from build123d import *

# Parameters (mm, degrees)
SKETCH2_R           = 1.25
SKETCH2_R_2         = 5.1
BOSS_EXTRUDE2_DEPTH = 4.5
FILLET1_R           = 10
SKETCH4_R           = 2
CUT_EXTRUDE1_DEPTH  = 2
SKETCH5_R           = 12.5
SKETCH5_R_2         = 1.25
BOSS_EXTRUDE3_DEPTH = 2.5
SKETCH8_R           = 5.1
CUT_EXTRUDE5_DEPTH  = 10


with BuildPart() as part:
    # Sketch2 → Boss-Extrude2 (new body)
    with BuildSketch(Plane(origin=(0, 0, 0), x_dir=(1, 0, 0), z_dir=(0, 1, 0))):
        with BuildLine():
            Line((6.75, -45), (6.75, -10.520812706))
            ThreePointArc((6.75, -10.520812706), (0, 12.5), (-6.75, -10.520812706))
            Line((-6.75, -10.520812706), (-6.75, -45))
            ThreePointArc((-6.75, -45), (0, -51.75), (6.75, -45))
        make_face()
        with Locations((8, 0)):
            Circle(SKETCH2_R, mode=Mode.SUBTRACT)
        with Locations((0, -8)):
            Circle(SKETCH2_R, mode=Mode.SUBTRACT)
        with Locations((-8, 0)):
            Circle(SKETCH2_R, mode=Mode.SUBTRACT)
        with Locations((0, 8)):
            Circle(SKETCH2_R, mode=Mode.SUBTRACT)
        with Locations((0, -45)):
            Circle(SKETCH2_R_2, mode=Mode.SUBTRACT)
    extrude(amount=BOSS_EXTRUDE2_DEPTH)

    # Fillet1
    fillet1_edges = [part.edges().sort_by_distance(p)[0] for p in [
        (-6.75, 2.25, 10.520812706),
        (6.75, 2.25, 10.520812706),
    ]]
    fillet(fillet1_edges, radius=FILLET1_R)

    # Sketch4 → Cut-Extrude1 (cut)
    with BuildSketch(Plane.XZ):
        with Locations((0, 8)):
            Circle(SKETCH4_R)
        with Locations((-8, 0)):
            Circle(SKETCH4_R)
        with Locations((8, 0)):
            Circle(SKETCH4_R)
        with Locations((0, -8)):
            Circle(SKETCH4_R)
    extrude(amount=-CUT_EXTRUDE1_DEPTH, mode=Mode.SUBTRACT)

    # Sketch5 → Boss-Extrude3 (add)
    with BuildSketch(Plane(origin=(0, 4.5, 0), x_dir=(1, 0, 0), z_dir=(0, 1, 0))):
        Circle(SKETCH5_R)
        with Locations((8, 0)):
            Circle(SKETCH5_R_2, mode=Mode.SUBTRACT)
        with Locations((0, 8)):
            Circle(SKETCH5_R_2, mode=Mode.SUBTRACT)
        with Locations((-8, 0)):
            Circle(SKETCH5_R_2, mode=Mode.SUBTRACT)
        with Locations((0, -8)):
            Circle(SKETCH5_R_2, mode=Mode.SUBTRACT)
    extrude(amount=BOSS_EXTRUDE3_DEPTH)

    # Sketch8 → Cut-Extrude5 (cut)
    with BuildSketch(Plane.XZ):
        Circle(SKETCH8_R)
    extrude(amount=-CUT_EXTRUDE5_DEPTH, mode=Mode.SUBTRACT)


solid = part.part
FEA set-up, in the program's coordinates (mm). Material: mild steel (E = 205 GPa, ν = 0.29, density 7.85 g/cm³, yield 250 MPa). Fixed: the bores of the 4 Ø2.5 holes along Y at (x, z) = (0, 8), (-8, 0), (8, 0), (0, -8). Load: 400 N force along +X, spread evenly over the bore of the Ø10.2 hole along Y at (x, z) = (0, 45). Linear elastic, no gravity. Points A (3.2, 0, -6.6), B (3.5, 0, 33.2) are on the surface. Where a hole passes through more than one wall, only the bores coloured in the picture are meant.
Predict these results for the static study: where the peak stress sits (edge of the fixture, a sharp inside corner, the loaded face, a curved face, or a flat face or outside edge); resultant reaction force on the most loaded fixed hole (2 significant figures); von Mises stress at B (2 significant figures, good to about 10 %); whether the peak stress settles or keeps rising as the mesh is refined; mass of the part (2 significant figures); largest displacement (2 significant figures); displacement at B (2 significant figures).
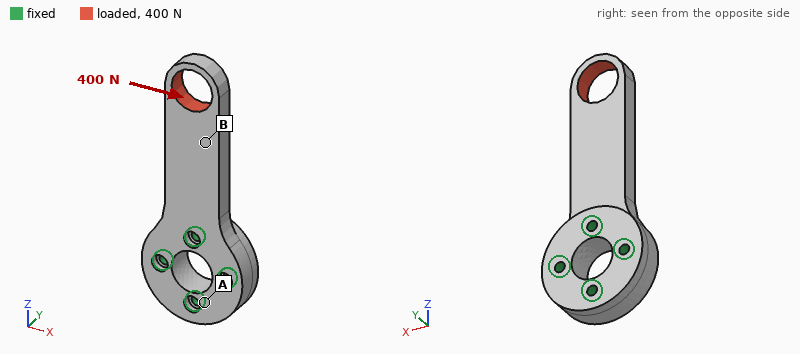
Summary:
edge of the fixture
870 N
19 MPa
keeps rising
37 g
63 µm
22 µm
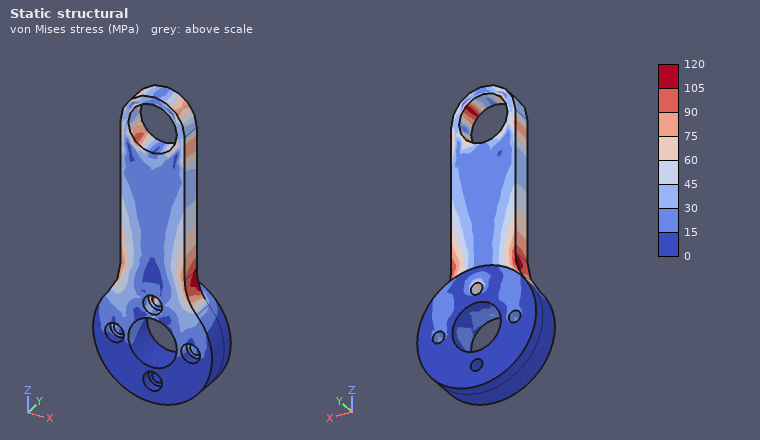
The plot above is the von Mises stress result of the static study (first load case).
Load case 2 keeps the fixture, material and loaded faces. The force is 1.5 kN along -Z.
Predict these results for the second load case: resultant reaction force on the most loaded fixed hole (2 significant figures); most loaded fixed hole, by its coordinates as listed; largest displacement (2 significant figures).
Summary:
850 N
(0, 8)
17 µm
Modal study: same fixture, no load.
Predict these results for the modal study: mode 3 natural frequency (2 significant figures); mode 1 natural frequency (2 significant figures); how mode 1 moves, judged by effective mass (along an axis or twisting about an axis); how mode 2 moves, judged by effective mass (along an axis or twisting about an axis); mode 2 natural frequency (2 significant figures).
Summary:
12 kHz
2800 Hz
along Y
along X
7000 Hz
